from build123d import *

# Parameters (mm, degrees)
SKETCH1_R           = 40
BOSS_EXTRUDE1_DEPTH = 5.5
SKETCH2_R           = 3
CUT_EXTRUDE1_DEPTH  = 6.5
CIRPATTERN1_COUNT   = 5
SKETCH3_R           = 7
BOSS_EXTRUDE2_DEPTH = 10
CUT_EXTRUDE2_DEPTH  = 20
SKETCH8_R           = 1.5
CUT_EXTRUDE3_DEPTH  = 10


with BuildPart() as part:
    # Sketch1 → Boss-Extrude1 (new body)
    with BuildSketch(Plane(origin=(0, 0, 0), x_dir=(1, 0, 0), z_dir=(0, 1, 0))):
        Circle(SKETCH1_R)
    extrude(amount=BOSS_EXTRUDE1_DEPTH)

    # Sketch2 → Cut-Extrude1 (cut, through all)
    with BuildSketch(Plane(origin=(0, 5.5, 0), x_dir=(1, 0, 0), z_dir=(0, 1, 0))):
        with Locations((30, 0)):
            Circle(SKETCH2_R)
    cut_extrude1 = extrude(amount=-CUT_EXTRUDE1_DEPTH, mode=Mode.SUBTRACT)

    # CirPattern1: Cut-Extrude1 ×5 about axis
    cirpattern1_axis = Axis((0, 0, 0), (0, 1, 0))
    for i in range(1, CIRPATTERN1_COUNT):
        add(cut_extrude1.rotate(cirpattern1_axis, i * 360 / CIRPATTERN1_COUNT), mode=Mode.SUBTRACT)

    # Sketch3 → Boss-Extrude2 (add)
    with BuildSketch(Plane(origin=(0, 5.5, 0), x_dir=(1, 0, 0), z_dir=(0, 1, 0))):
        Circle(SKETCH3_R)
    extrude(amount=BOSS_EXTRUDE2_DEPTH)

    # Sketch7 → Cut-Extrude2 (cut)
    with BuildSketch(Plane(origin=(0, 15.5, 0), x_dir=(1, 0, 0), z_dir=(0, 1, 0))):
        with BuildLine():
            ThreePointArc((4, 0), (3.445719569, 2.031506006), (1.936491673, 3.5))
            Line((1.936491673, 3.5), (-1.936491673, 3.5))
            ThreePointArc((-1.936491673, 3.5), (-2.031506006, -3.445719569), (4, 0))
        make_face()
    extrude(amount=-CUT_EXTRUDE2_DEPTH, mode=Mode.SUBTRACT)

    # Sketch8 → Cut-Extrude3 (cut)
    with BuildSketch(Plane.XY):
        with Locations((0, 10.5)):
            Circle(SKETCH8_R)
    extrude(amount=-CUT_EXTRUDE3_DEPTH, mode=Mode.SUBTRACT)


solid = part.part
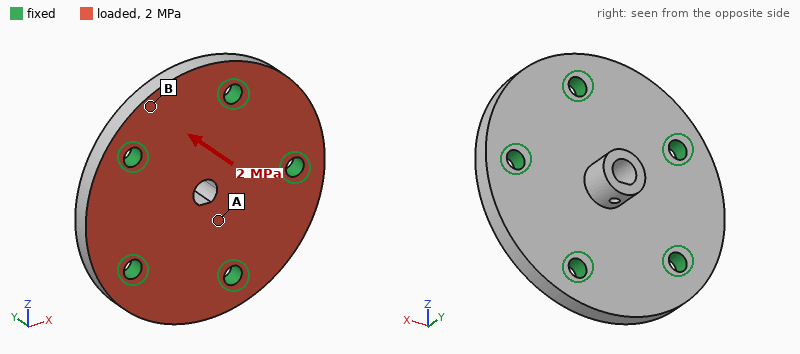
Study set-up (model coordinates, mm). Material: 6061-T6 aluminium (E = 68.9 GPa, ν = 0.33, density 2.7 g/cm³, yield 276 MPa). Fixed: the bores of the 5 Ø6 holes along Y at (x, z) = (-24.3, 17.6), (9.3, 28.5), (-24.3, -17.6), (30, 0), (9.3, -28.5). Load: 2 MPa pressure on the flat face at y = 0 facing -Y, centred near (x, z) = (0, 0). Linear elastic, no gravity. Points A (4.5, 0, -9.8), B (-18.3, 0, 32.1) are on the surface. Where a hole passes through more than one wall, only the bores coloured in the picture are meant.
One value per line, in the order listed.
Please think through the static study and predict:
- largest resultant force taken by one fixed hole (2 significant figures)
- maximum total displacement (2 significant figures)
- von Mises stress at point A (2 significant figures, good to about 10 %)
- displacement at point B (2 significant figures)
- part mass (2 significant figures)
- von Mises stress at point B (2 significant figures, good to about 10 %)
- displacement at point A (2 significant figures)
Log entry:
1.9 kN
26 µm
17 MPa
12 µm
75 g
11 MPa
22 µm
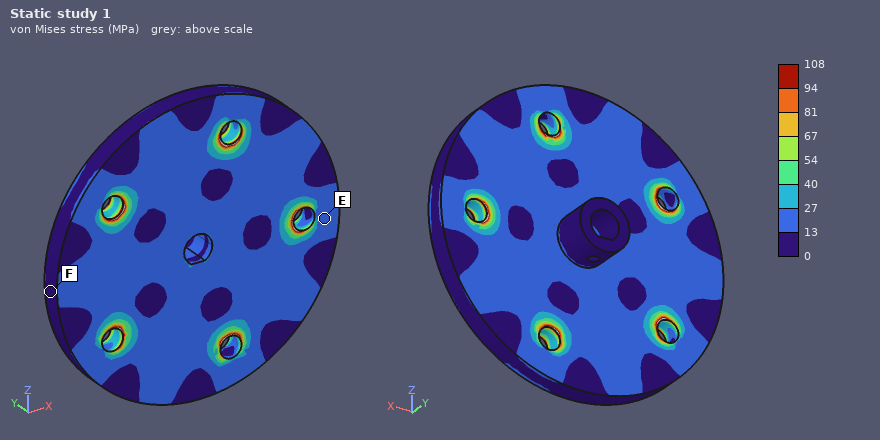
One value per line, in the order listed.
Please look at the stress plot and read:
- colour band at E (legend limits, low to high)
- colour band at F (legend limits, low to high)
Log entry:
13 to 27 MPa
0 to 13 MPa
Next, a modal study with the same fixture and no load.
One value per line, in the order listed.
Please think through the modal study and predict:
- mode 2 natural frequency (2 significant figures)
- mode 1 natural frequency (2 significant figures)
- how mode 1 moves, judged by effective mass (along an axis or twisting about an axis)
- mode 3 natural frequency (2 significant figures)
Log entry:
16 kHz
12 kHz
along Y
16 kHz
